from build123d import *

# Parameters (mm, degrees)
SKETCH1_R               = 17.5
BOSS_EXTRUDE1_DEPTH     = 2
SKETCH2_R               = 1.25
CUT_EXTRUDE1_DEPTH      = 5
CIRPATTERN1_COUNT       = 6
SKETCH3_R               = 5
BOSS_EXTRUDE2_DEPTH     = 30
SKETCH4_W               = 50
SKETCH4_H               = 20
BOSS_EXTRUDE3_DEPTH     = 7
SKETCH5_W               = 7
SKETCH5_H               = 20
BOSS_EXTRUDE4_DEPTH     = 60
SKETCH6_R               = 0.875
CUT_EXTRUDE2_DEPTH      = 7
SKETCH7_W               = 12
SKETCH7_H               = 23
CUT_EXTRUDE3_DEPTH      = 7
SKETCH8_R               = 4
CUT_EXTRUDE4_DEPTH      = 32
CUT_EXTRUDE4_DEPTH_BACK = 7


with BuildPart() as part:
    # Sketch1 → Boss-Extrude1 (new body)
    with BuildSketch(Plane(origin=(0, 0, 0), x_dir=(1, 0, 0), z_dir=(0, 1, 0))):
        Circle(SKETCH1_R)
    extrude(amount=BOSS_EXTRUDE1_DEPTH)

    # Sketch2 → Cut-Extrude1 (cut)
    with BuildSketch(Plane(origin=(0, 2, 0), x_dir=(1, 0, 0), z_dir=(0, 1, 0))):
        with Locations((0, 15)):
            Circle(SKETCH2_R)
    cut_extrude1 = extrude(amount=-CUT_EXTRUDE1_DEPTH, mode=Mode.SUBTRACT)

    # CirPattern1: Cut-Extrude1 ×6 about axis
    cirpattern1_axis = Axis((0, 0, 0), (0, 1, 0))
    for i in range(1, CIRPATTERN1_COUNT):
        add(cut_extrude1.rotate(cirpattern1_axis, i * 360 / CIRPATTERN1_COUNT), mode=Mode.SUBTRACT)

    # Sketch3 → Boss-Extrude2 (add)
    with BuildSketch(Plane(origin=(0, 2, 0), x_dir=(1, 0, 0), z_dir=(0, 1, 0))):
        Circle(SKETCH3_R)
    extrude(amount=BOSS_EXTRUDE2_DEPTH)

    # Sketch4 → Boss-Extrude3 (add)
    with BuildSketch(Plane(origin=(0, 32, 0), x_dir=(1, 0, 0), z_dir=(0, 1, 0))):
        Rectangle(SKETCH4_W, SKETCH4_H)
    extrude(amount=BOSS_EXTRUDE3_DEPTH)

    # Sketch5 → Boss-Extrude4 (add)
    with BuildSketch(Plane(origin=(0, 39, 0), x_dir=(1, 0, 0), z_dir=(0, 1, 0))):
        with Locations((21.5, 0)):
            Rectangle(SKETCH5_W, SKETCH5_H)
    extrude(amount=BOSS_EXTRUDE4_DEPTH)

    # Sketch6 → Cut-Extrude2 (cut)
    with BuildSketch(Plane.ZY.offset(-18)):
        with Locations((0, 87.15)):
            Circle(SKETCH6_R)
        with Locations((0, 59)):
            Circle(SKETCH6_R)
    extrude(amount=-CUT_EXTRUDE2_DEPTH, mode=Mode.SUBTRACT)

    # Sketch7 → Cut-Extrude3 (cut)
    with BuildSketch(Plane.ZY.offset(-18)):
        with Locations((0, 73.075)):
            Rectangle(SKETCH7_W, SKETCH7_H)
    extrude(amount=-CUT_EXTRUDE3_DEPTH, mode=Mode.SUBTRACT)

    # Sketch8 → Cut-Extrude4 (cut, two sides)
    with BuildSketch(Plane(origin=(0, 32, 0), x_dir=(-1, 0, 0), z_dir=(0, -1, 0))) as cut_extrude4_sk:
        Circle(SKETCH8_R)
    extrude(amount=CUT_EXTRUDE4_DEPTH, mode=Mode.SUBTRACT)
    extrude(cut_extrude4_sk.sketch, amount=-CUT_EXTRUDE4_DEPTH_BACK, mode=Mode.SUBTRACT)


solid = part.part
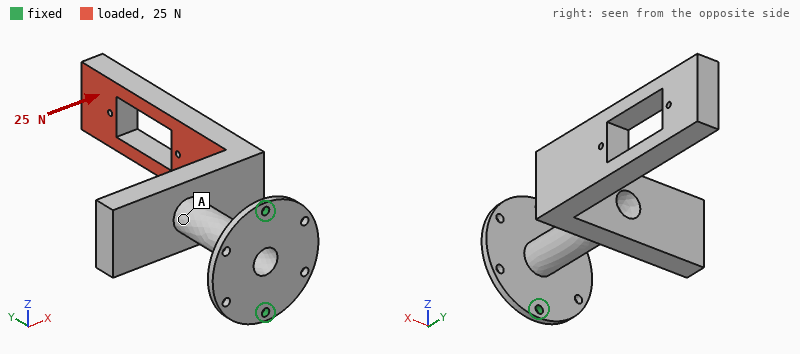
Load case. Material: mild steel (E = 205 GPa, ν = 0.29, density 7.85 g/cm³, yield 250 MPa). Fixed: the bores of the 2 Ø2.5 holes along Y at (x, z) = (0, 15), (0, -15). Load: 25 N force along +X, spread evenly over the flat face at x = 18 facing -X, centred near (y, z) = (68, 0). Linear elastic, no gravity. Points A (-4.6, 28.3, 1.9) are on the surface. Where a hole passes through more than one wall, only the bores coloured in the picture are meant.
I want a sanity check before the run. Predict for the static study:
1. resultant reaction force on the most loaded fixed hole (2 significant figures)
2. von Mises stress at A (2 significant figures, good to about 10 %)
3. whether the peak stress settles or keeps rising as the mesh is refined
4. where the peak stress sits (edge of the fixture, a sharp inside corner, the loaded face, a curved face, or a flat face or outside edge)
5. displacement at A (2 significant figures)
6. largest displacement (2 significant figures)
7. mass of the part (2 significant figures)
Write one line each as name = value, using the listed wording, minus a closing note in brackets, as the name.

resultant reaction force on the most loaded fixed hole = 13 N
von Mises stress at A = 15 MPa
whether the peak stress settles or keeps rising as the mesh is refined = keeps rising
where the peak stress sits = edge of the fixture
displacement at A = 0.082 mm
largest displacement = 0.34 mm
mass of the part = 120 g
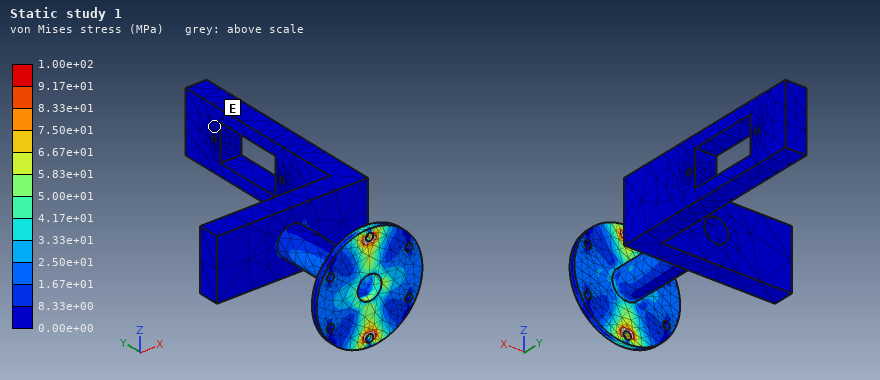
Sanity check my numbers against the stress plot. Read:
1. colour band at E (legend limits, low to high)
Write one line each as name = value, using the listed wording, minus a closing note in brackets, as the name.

colour band at E = 0.00e+00 to 8.33e+00 MPa
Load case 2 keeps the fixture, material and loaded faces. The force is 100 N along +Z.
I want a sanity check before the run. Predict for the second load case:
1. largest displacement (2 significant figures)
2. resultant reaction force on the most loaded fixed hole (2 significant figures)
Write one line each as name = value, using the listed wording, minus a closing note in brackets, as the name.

largest displacement = 0.60 mm
resultant reaction force on the most loaded fixed hole = 310 N
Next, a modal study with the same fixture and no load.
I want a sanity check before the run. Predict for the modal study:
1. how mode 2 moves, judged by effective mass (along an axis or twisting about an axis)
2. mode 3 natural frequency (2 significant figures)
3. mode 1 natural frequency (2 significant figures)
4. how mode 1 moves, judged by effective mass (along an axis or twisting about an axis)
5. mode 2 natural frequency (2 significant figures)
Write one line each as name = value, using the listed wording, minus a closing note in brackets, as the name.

how mode 2 moves, judged by effective mass = along Z
mode 3 natural frequency = 1300 Hz
mode 1 natural frequency = 190 Hz
how mode 1 moves, judged by effective mass = along X
mode 2 natural frequency = 310 Hz
